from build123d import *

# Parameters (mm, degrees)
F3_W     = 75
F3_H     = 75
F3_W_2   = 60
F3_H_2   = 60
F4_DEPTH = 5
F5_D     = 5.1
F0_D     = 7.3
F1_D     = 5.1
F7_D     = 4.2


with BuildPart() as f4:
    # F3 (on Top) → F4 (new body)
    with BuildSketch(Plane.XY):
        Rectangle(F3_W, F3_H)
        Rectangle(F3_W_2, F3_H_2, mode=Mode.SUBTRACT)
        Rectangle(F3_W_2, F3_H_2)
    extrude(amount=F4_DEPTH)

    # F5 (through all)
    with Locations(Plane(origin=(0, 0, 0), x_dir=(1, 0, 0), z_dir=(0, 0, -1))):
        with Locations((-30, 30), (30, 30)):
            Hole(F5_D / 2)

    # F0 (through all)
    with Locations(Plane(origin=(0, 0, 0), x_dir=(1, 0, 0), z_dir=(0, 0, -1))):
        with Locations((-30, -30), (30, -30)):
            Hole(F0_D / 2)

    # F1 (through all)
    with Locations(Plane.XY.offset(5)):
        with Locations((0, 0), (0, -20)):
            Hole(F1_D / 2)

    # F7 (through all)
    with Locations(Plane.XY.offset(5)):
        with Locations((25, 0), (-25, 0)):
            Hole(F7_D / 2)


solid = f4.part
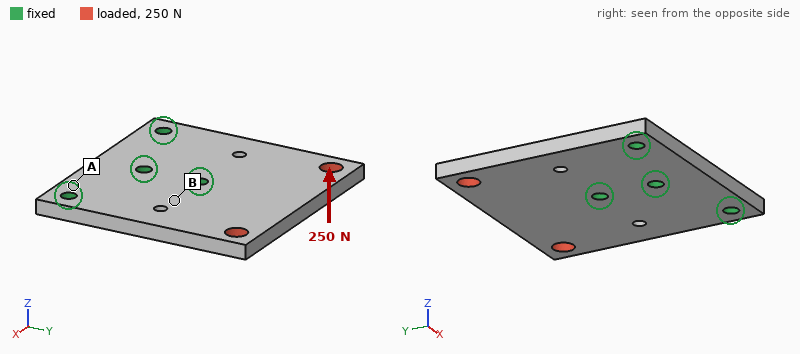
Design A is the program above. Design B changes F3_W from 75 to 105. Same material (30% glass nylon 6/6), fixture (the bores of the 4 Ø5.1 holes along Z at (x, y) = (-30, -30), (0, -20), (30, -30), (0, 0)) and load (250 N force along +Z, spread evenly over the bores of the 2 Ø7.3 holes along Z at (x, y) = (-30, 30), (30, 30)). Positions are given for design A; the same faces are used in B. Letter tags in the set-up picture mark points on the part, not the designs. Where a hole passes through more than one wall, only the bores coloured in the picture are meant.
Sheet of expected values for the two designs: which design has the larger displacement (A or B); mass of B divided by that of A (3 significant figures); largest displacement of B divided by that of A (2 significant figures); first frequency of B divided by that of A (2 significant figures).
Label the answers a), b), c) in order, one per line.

a) A
b) 1.41
c) 0.91
d) 0.71
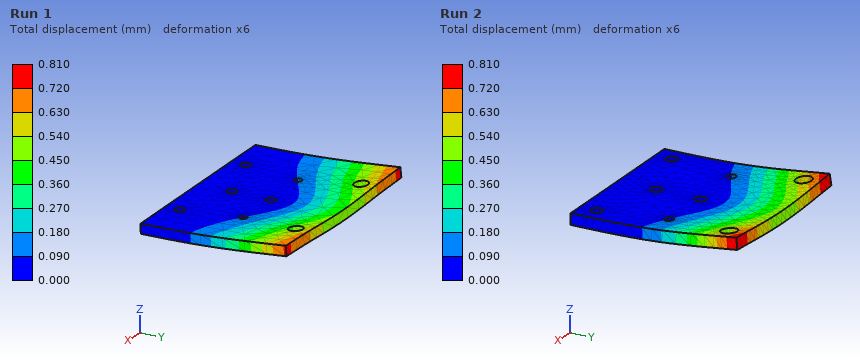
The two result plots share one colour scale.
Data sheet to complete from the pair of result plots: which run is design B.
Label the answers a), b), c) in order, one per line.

a) Run 1
